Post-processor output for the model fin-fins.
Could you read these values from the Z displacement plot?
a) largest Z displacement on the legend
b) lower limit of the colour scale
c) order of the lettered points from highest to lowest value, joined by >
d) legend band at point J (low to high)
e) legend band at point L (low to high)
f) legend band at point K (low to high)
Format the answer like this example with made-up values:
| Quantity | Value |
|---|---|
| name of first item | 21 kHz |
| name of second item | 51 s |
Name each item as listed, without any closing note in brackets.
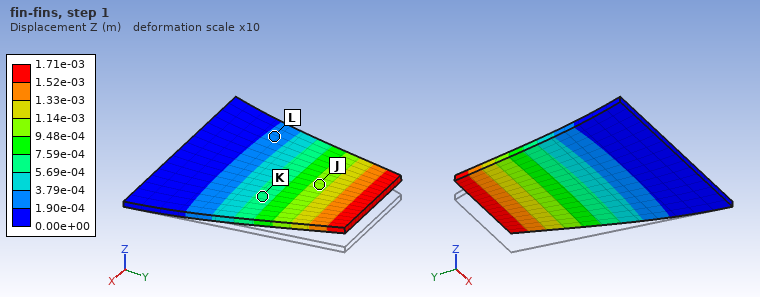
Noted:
| Quantity | Value |
|---|---|
| largest Z displacement on the legend | 1.71e-03 m |
| lower limit of the colour scale | 0.00e+00 m |
| order of the lettered points from highest to lowest value, joined by > | J > K > L |
| legend band at point J | 9.48e-04 to 1.14e-03 m |
| legend band at point L | 1.90e-04 to 3.79e-04 m |
| legend band at point K | 5.69e-04 to 7.59e-04 m |
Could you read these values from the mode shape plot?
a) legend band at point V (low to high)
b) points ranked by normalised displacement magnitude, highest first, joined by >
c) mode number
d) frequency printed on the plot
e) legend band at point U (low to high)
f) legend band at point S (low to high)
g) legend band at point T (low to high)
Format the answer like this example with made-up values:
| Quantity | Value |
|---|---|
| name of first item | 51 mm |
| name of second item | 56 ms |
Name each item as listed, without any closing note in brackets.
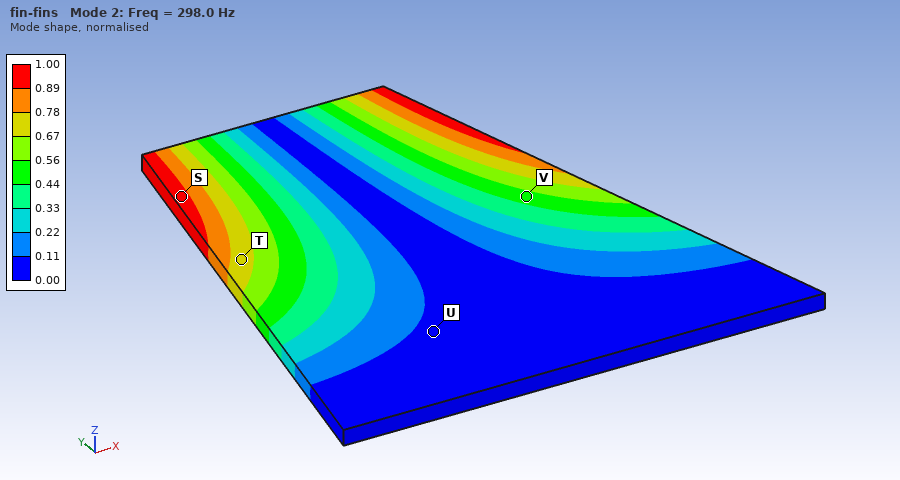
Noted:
| Quantity | Value |
|---|---|
| legend band at point V | 0.44 to 0.56 |
| points ranked by normalised displacement magnitude, highest first, joined by > | S > T > V > U |
| mode number | 2 |
| frequency printed on the plot | 298.0 Hz |
| legend band at point U | 0.00 to 0.11 |
| legend band at point S | 0.89 to 1.00 |
| legend band at point T | 0.67 to 0.78 |
